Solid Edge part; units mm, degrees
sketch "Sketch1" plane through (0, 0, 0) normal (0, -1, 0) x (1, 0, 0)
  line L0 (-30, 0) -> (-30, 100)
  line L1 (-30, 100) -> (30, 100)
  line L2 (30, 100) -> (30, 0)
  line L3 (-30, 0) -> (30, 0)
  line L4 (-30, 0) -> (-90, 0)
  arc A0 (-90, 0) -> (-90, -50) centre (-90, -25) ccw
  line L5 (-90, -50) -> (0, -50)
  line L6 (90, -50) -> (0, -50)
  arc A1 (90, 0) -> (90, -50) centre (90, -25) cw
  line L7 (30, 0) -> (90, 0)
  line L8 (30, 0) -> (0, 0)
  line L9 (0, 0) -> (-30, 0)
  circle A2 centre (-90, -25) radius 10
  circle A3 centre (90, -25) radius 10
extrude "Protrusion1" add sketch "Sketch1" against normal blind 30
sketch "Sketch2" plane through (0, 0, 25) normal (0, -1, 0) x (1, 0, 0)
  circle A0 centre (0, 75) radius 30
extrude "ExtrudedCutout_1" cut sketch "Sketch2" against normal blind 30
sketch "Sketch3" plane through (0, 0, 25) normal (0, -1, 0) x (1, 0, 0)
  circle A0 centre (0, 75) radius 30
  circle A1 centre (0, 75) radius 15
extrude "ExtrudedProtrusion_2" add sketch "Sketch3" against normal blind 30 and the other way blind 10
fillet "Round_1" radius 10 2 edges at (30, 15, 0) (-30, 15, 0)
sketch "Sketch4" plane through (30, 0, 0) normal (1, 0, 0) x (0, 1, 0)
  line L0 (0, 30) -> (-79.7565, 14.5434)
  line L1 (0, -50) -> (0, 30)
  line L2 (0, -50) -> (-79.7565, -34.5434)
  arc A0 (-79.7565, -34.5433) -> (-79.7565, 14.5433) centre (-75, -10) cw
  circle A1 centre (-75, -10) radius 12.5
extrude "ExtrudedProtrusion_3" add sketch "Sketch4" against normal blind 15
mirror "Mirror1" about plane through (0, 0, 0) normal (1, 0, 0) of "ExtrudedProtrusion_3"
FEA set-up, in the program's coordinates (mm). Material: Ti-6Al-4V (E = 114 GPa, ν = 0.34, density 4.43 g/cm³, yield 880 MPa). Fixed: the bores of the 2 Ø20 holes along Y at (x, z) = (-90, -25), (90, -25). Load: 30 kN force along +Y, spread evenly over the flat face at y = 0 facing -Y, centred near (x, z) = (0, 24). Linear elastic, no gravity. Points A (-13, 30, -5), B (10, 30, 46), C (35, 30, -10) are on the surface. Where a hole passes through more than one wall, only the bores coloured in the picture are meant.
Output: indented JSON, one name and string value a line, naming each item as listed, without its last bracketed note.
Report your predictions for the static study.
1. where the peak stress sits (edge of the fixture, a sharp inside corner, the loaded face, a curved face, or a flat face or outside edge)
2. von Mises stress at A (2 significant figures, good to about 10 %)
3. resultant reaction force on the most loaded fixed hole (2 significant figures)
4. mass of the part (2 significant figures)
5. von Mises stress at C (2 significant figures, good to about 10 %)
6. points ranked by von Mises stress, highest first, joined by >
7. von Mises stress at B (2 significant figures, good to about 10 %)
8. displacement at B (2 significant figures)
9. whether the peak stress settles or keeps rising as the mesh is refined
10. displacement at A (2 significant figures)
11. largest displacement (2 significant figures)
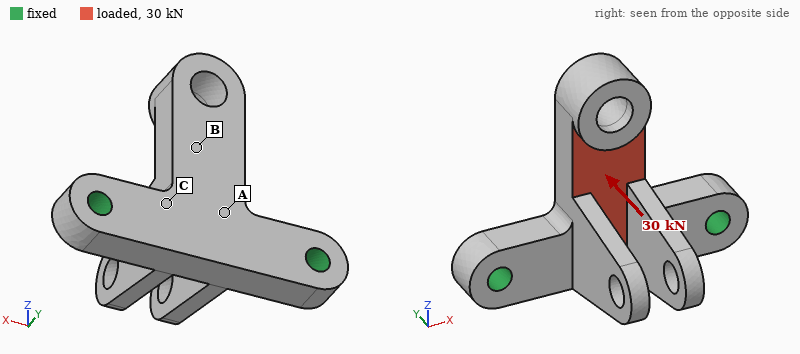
{
  "where the peak stress sits": "edge of the fixture",
  "von Mises stress at A": "74 MPa",
  "resultant reaction force on the most loaded fixed hole": "15 kN",
  "mass of the part": "3.1 kg",
  "von Mises stress at C": "110 MPa",
  "points ranked by von Mises stress, highest first, joined by >": "C > A > B",
  "von Mises stress at B": "25 MPa",
  "displacement at B": "0.36 mm",
  "whether the peak stress settles or keeps rising as the mesh is refined": "keeps rising",
  "displacement at A": "0.15 mm",
  "largest displacement": "0.79 mm"
}
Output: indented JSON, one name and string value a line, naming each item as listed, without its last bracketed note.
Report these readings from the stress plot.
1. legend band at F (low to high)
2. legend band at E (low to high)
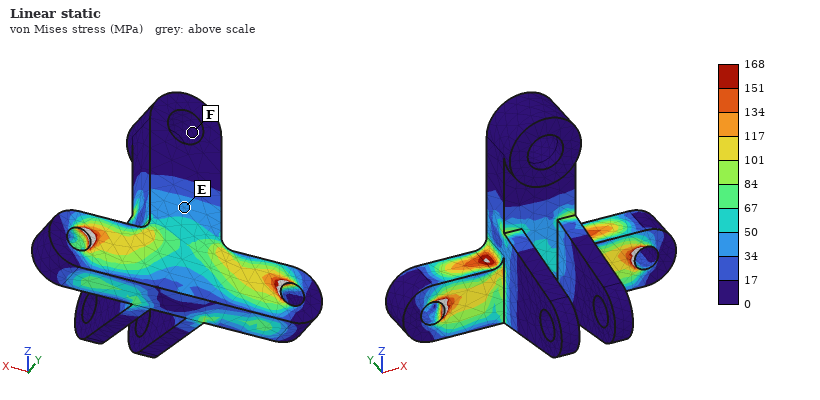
{
  "legend band at F": "0 to 17 MPa",
  "legend band at E": "34 to 50 MPa"
}
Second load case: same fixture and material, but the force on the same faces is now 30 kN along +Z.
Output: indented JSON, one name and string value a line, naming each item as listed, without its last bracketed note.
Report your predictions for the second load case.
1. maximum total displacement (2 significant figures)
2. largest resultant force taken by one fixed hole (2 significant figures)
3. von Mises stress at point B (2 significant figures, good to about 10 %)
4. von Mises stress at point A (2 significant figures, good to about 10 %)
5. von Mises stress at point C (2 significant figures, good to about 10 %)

{
  "maximum total displacement": "0.26 mm",
  "largest resultant force taken by one fixed hole": "15 kN",
  "von Mises stress at point B": "12 MPa",
  "von Mises stress at point A": "26 MPa",
  "von Mises stress at point C": "16 MPa"
}
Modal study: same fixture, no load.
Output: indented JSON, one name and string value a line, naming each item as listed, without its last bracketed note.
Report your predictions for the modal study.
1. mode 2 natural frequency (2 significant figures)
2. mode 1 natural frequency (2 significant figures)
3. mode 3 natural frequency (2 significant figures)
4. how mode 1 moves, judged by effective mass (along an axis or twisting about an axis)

{
  "mode 2 natural frequency": "1500 Hz",
  "mode 1 natural frequency": "810 Hz",
  "mode 3 natural frequency": "1500 Hz",
  "how mode 1 moves, judged by effective mass": "along Y"
}
